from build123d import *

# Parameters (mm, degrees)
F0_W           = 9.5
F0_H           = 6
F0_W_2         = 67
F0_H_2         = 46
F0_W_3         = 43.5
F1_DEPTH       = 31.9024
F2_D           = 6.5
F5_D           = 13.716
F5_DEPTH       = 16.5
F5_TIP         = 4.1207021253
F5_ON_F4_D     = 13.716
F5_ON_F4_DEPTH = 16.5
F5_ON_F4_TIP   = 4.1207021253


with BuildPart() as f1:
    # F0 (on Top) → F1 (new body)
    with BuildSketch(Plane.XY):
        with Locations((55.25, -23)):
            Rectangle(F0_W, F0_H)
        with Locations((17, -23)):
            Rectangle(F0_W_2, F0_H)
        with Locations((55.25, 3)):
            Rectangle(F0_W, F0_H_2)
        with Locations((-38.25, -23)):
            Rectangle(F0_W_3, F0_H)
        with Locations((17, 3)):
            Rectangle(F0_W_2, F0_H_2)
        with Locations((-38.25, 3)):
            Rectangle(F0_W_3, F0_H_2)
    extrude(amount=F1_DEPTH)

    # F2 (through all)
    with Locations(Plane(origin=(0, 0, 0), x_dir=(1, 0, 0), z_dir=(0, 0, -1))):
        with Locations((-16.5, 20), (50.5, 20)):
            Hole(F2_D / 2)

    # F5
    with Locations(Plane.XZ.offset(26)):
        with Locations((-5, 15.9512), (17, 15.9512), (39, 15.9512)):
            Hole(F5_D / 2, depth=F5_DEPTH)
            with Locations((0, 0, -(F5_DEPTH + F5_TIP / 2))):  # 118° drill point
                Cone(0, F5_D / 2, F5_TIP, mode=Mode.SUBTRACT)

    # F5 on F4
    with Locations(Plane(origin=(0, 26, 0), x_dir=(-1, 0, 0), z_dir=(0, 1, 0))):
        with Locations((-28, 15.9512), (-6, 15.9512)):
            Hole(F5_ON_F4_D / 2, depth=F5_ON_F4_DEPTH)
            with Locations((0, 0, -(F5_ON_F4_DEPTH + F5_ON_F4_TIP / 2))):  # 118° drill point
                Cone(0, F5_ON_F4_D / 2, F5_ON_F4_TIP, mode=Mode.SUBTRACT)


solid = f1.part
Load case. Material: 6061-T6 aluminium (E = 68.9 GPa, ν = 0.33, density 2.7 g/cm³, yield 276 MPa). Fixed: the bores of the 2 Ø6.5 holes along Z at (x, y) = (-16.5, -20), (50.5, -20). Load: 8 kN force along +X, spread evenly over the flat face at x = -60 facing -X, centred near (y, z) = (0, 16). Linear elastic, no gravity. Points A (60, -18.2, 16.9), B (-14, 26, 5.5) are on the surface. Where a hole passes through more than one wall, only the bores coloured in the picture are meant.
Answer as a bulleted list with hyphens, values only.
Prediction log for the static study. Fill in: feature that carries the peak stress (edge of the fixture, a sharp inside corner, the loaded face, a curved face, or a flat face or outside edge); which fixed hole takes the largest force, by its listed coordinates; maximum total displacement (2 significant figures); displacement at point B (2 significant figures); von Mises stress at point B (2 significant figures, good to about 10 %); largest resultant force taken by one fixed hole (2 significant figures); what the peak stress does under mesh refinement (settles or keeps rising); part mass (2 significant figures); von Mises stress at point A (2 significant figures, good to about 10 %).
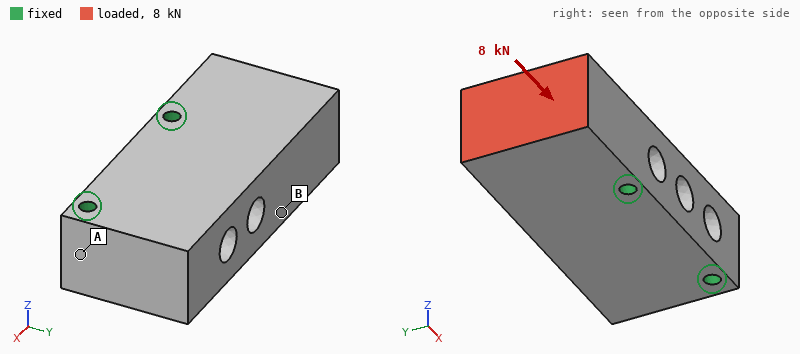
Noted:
- edge of the fixture
- (-16.5, -20)
- 14 µm
- 7.7 µm
- 6.7 MPa
- 5.8 kN
- keeps rising
- 500 g
- 3.3 MPa
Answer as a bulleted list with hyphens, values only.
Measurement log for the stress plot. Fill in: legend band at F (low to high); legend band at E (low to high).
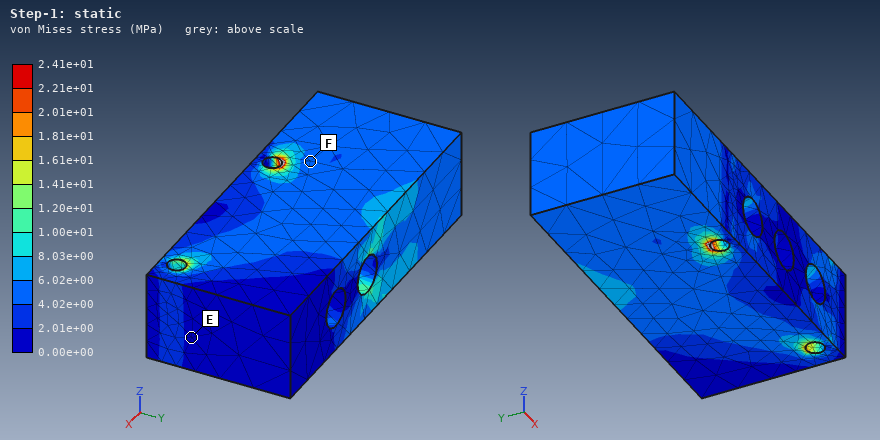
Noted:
- 4.02e+00 to 6.02e+00 MPa
- 0.00e+00 to 2.01e+00 MPa
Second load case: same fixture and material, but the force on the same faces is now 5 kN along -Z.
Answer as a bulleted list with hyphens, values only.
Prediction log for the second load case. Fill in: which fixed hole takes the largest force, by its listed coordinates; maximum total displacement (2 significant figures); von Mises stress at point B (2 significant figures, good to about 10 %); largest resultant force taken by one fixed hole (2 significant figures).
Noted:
- (-16.5, -20)
- 48 µm
- 7.2 MPa
- 5.9 kN
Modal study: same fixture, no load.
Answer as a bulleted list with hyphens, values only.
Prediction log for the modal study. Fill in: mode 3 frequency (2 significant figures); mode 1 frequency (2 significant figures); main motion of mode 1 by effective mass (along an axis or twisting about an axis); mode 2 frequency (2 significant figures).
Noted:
- 7500 Hz
- 5500 Hz
- along Z
- 7100 Hz
